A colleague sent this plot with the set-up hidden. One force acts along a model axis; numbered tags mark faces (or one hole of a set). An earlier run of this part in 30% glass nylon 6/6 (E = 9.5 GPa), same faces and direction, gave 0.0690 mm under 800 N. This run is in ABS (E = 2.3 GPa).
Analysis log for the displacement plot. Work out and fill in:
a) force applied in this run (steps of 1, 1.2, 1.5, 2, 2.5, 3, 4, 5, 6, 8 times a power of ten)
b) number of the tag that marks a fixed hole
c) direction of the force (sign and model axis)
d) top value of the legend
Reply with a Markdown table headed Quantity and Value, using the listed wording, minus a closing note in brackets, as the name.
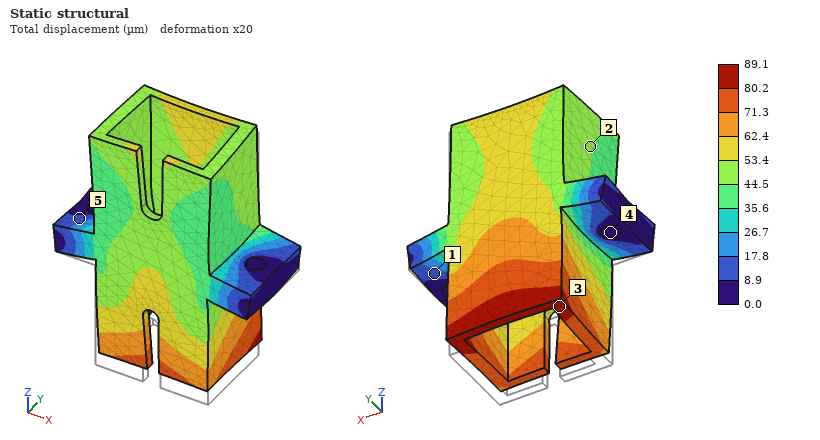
| Quantity | Value |
|---|---|
| force applied in this run | 250 N |
| number of the tag that marks a fixed hole | 4 |
| direction of the force | +Z |
| top value of the legend | 89.1 µm |
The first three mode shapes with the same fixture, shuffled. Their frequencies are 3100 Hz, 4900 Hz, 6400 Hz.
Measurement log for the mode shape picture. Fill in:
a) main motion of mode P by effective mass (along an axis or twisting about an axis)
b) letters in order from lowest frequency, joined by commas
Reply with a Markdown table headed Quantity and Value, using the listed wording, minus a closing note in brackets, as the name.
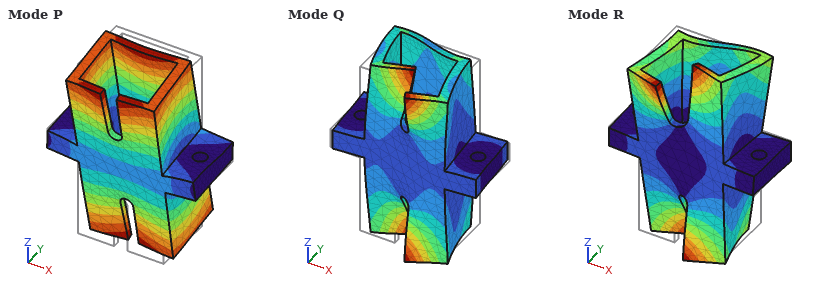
| Quantity | Value |
|---|---|
| main motion of mode P by effective mass | twisting about X |
| letters in order from lowest frequency, joined by commas | P, R, Q |
